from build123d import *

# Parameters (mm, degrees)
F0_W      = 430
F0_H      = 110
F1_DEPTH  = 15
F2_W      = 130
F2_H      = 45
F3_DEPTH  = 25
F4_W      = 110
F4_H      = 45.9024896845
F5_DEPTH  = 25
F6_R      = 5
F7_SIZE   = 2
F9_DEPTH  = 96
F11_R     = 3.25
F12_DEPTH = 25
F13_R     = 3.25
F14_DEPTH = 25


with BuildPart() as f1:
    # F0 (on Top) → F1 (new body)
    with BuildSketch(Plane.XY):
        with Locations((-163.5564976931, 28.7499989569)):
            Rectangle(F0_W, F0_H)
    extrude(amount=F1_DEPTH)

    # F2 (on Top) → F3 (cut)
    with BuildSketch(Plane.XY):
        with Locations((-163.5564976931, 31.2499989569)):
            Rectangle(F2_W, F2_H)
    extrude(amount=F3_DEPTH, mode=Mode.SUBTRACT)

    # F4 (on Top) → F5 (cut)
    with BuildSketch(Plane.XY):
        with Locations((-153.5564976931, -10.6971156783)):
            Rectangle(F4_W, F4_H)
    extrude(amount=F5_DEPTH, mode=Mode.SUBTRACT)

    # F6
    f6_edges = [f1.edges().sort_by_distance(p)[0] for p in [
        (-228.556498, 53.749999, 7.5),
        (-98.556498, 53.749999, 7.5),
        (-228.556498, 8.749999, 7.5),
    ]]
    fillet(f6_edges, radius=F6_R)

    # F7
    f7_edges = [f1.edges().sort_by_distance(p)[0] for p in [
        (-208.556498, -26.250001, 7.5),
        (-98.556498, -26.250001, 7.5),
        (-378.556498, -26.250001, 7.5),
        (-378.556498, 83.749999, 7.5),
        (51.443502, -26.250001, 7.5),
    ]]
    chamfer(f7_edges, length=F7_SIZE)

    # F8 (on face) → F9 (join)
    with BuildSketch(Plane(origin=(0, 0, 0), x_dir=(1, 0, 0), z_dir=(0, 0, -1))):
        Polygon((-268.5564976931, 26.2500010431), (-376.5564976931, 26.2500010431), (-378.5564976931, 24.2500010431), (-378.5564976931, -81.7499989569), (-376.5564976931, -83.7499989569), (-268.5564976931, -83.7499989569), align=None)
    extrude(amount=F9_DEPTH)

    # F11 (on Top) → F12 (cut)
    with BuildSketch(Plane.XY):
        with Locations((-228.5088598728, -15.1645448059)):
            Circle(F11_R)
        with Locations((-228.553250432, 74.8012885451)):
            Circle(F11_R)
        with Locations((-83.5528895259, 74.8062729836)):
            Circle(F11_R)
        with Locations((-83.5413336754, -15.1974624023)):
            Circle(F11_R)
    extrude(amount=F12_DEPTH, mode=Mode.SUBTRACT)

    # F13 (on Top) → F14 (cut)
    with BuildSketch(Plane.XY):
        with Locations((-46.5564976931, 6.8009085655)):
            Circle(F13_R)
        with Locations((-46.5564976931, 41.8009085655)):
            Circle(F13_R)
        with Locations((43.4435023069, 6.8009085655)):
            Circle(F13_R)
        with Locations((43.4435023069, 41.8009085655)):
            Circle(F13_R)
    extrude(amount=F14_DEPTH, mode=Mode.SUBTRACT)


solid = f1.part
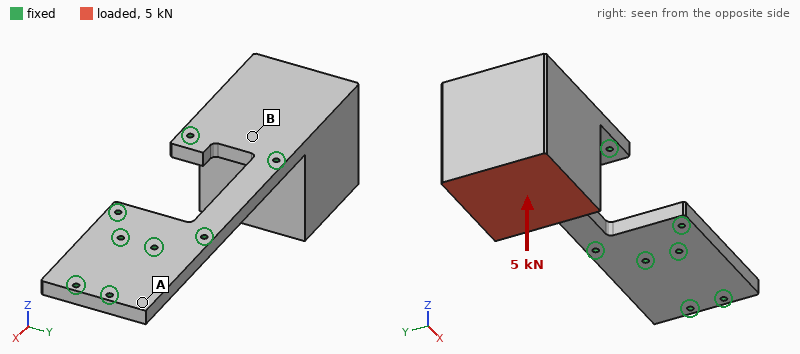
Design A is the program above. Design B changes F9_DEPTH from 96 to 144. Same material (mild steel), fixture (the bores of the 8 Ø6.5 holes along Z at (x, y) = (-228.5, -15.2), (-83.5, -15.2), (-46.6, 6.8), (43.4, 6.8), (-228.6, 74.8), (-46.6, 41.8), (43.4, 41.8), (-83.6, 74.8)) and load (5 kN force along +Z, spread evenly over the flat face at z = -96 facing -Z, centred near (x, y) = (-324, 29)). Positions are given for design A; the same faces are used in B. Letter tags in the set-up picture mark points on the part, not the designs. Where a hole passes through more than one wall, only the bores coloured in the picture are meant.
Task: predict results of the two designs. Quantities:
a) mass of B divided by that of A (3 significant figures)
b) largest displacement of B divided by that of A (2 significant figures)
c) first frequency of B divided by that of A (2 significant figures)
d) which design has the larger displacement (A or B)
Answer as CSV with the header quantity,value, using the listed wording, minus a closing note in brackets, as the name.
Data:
quantity,value
mass of B divided by that of A,1.34
largest displacement of B divided by that of A,1.2
first frequency of B divided by that of A,0.71
which design has the larger displacement,B
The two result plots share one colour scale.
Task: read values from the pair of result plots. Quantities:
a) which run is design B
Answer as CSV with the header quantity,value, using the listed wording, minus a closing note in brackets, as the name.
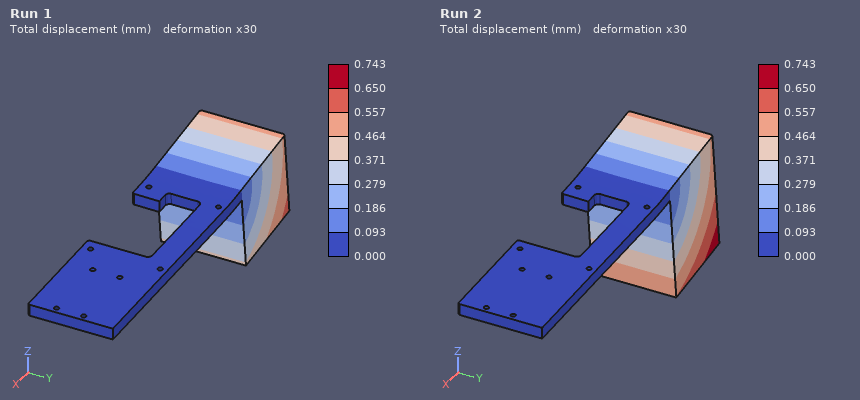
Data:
quantity,value
which run is design B,Run 2
